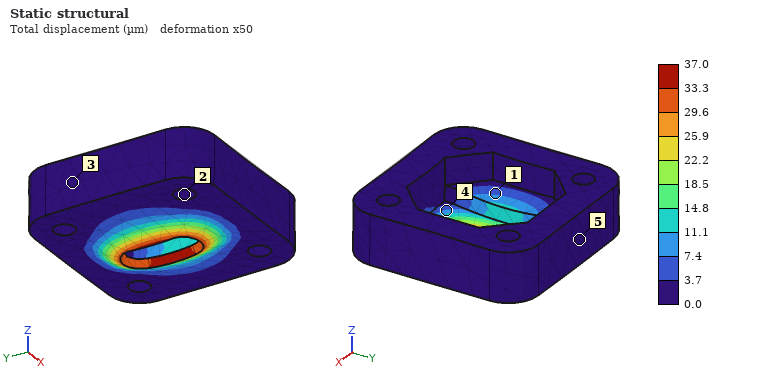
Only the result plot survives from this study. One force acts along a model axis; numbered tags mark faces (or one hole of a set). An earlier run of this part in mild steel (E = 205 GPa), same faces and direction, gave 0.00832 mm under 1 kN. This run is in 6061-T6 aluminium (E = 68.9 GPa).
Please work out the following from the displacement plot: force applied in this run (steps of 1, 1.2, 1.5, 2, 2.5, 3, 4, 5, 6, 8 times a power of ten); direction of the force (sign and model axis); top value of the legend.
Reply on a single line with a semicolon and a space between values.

1.5 kN; -Z; 37.0 µm
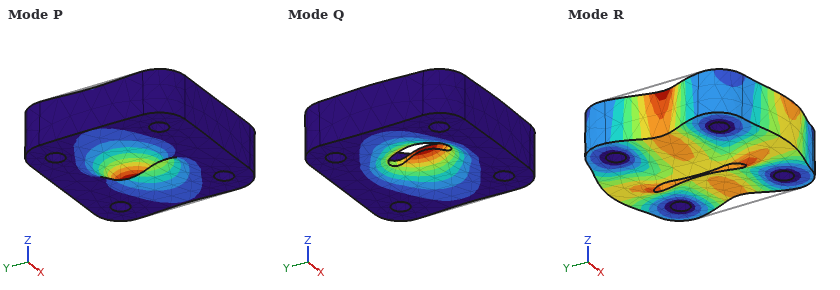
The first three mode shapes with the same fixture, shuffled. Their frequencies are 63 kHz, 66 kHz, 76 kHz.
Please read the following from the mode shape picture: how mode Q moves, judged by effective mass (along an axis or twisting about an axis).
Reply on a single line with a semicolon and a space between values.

along Z
